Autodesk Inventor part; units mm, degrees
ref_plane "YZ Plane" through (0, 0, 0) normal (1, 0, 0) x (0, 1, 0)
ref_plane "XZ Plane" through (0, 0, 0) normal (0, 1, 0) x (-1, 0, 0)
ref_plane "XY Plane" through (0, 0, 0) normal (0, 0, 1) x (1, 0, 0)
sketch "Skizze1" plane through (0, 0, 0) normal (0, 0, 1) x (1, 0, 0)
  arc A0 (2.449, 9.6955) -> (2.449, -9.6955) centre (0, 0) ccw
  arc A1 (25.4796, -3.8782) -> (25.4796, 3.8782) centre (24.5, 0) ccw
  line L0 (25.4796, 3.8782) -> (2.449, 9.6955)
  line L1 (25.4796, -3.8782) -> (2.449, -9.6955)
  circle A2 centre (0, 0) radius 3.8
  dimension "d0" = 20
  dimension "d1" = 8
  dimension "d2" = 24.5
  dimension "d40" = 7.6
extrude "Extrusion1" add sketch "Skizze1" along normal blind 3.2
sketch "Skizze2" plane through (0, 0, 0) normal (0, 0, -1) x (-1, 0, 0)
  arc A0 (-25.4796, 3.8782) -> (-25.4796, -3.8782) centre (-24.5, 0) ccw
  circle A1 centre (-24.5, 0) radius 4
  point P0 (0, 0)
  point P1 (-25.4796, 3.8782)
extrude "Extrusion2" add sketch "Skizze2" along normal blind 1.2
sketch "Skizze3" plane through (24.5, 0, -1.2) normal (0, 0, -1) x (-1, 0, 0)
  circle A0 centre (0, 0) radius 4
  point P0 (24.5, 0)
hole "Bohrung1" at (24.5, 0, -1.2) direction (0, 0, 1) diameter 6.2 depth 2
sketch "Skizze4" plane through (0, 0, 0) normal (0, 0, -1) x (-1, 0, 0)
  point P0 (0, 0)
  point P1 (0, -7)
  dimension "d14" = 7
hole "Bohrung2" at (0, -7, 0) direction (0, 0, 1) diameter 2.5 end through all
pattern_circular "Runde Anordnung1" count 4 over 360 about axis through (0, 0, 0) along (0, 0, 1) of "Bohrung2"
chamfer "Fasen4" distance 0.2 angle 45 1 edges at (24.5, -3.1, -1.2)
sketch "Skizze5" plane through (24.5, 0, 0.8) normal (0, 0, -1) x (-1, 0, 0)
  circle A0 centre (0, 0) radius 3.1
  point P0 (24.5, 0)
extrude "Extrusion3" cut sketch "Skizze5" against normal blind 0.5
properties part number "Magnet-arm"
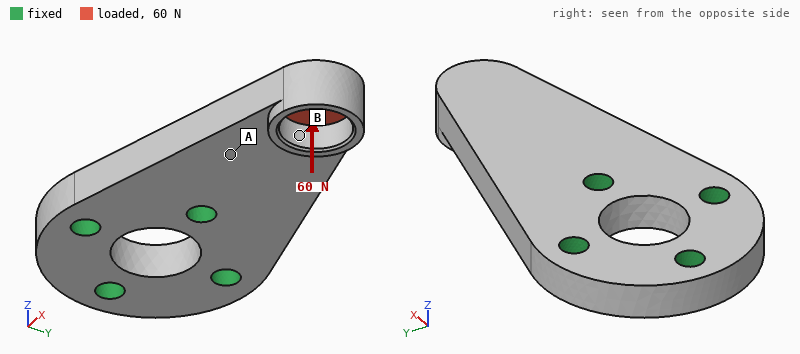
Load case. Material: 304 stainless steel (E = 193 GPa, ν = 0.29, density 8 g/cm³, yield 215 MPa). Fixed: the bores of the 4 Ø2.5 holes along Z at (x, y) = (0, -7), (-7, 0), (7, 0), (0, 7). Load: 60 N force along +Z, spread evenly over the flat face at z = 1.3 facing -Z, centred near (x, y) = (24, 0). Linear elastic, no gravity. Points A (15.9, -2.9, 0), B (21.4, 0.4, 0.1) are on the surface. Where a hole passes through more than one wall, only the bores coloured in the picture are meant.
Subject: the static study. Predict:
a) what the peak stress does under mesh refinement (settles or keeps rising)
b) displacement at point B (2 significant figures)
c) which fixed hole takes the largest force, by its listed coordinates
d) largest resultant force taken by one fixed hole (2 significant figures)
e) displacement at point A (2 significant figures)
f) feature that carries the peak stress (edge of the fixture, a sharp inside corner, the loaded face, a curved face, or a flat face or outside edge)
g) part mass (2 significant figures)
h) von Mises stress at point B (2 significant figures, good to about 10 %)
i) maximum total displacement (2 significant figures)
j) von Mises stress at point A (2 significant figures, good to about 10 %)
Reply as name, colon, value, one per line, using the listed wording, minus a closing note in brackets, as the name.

what the peak stress does under mesh refinement: keeps rising
displacement at point B: 11 µm
which fixed hole takes the largest force, by its listed coordinates: (7, 0)
largest resultant force taken by one fixed hole: 120 N
displacement at point A: 5.0 µm
feature that carries the peak stress: edge of the fixture
part mass: 12 g
von Mises stress at point B: 7.9 MPa
maximum total displacement: 21 µm
von Mises stress at point A: 23 MPa
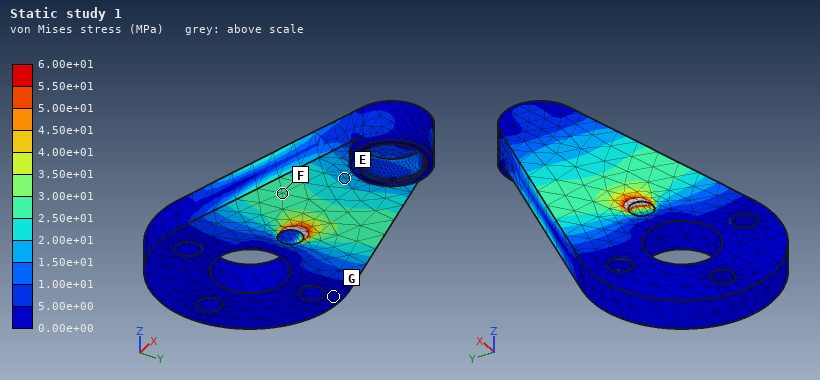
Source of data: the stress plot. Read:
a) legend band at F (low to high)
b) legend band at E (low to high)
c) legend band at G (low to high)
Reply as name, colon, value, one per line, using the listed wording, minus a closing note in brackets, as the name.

legend band at F: 2.50e+01 to 3.00e+01 MPa
legend band at E: 1.50e+01 to 2.00e+01 MPa
legend band at G: 0.00e+00 to 5.00e+00 MPa
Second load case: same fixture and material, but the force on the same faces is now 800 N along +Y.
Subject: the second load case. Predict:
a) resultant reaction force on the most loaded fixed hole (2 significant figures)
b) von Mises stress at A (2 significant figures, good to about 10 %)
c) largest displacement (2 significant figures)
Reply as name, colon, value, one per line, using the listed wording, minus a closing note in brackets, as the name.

resultant reaction force on the most loaded fixed hole: 870 N
von Mises stress at A: 55 MPa
largest displacement: 29 µm
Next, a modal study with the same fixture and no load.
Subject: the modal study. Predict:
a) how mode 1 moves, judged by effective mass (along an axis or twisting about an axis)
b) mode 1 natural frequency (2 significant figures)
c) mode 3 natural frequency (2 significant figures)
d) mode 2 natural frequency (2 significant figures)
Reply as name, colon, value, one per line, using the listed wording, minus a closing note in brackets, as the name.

how mode 1 moves, judged by effective mass: along Z
mode 1 natural frequency: 7500 Hz
mode 3 natural frequency: 23 kHz
mode 2 natural frequency: 22 kHz
